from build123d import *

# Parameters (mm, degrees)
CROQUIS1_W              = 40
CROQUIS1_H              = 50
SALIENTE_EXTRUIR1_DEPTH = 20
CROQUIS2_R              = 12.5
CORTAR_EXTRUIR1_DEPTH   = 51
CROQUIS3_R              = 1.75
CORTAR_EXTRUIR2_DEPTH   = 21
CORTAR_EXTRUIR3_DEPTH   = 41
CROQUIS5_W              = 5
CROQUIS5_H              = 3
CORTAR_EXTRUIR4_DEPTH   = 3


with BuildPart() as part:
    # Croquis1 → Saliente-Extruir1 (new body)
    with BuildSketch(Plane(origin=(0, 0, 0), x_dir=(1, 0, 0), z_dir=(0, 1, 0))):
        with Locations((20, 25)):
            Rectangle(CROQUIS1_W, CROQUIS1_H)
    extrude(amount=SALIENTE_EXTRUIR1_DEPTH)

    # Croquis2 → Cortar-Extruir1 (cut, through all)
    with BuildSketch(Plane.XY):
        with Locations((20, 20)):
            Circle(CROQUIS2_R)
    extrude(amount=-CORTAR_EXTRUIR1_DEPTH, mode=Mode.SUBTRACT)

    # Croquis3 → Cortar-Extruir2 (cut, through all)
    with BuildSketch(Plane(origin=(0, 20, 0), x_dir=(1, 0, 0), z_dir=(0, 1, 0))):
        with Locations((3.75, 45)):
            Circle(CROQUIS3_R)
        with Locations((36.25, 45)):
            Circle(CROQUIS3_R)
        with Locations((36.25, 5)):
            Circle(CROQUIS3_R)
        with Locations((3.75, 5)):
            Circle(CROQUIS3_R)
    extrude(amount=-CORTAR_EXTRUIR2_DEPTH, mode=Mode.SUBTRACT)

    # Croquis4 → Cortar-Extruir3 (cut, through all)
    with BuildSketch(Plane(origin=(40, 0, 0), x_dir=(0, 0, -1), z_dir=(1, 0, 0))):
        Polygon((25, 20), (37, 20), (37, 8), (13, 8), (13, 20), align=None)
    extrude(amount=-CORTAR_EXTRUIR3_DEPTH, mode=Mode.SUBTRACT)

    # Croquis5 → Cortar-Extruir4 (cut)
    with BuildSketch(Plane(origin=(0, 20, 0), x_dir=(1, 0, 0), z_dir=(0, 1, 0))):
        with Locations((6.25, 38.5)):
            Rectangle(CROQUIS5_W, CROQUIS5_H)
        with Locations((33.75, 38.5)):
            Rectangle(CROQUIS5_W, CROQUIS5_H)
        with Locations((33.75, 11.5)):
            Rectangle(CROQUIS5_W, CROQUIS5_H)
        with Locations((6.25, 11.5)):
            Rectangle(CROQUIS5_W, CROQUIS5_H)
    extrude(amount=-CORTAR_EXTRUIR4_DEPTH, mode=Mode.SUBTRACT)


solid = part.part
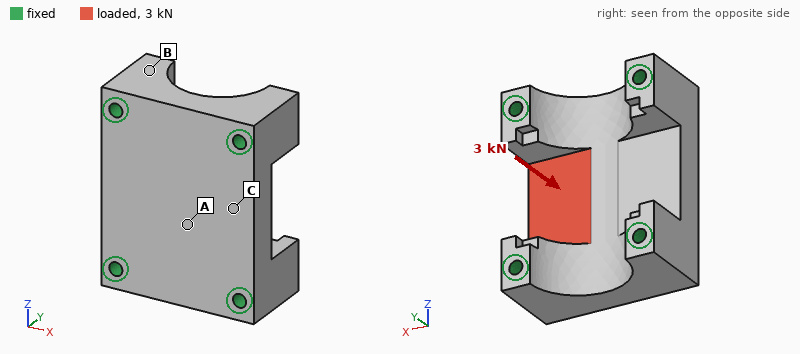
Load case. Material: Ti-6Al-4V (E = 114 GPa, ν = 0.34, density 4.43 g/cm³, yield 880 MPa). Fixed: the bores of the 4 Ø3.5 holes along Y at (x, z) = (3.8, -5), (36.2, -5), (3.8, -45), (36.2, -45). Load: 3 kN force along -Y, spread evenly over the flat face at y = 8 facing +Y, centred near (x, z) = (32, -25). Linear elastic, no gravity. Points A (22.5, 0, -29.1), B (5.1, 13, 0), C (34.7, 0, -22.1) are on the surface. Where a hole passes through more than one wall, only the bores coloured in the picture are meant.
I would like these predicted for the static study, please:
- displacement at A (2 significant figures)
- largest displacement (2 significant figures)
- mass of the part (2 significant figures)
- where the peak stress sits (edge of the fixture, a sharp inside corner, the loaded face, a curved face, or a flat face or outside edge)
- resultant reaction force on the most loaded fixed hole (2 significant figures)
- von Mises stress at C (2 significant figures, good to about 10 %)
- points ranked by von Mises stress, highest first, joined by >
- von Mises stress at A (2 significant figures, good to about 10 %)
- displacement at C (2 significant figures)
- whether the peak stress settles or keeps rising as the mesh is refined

4.1 µm
8.3 µm
94 g
edge of the fixture
1.4 kN
26 MPa
C > A > B
14 MPa
6.5 µm
keeps rising
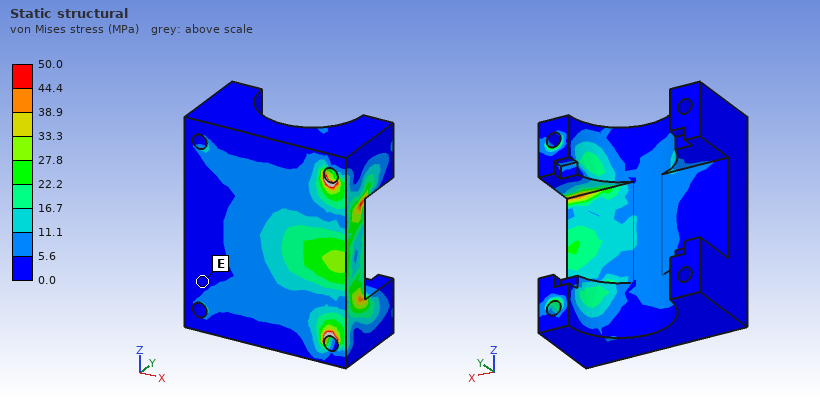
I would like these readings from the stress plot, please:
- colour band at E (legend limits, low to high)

0.0 to 5.6 MPa
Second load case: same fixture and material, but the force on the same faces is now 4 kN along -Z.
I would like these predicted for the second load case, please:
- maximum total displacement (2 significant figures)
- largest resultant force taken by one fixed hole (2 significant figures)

2.9 µm
1.6 kN
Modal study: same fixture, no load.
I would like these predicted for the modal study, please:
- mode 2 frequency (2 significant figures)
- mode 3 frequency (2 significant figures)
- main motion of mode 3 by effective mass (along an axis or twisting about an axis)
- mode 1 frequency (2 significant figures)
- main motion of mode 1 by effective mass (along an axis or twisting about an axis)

32 kHz
35 kHz
along X
24 kHz
along Y
